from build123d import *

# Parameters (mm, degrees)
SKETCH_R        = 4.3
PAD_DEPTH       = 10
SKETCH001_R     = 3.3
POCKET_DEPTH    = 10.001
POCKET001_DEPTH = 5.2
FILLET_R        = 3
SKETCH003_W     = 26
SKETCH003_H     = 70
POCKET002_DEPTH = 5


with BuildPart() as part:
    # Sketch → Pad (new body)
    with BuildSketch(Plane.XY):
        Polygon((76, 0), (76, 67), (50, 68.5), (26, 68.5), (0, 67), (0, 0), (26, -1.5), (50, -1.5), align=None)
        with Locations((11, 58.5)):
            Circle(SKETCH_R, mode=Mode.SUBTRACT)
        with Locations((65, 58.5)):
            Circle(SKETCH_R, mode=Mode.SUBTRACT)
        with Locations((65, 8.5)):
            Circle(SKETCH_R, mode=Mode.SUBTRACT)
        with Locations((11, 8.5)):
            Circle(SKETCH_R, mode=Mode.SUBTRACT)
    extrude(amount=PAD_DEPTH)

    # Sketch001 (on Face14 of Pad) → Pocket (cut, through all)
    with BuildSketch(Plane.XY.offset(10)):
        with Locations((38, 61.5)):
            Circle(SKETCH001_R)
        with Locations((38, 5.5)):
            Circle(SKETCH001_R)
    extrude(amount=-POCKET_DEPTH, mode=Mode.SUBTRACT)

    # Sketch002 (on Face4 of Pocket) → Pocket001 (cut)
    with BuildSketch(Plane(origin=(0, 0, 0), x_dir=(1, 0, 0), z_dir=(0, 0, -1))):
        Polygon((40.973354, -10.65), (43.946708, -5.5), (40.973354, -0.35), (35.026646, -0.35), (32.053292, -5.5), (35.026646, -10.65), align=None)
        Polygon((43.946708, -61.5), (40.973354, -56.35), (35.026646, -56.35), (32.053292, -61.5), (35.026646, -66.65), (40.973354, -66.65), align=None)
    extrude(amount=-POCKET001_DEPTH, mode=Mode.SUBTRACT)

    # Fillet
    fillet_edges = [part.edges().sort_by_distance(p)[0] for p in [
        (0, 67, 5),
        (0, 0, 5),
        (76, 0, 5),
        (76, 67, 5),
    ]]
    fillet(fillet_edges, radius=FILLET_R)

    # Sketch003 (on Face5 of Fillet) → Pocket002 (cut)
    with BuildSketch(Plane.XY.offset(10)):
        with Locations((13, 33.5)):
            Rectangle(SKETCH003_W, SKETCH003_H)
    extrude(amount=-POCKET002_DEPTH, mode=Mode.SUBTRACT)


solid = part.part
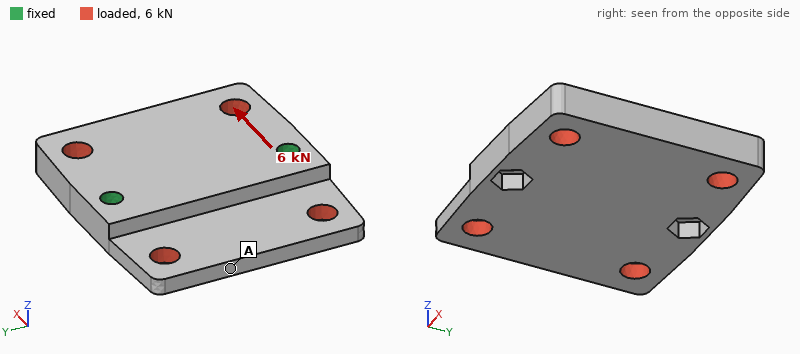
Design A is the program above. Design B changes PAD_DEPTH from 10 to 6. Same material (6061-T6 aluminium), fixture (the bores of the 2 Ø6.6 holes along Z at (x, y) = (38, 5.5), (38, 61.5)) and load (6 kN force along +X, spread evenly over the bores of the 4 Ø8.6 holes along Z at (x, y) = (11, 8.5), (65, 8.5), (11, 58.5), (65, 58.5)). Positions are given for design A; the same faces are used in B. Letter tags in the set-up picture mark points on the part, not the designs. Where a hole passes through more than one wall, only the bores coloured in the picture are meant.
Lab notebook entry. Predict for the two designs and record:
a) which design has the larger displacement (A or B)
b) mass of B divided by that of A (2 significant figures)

B
0.68
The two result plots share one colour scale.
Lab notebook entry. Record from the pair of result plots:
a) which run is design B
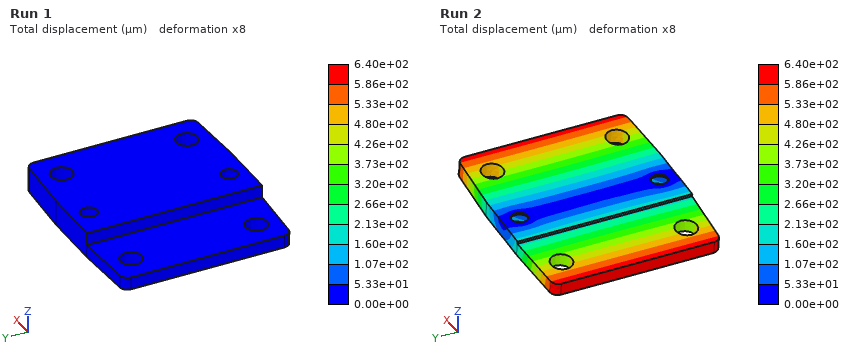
Run 2
